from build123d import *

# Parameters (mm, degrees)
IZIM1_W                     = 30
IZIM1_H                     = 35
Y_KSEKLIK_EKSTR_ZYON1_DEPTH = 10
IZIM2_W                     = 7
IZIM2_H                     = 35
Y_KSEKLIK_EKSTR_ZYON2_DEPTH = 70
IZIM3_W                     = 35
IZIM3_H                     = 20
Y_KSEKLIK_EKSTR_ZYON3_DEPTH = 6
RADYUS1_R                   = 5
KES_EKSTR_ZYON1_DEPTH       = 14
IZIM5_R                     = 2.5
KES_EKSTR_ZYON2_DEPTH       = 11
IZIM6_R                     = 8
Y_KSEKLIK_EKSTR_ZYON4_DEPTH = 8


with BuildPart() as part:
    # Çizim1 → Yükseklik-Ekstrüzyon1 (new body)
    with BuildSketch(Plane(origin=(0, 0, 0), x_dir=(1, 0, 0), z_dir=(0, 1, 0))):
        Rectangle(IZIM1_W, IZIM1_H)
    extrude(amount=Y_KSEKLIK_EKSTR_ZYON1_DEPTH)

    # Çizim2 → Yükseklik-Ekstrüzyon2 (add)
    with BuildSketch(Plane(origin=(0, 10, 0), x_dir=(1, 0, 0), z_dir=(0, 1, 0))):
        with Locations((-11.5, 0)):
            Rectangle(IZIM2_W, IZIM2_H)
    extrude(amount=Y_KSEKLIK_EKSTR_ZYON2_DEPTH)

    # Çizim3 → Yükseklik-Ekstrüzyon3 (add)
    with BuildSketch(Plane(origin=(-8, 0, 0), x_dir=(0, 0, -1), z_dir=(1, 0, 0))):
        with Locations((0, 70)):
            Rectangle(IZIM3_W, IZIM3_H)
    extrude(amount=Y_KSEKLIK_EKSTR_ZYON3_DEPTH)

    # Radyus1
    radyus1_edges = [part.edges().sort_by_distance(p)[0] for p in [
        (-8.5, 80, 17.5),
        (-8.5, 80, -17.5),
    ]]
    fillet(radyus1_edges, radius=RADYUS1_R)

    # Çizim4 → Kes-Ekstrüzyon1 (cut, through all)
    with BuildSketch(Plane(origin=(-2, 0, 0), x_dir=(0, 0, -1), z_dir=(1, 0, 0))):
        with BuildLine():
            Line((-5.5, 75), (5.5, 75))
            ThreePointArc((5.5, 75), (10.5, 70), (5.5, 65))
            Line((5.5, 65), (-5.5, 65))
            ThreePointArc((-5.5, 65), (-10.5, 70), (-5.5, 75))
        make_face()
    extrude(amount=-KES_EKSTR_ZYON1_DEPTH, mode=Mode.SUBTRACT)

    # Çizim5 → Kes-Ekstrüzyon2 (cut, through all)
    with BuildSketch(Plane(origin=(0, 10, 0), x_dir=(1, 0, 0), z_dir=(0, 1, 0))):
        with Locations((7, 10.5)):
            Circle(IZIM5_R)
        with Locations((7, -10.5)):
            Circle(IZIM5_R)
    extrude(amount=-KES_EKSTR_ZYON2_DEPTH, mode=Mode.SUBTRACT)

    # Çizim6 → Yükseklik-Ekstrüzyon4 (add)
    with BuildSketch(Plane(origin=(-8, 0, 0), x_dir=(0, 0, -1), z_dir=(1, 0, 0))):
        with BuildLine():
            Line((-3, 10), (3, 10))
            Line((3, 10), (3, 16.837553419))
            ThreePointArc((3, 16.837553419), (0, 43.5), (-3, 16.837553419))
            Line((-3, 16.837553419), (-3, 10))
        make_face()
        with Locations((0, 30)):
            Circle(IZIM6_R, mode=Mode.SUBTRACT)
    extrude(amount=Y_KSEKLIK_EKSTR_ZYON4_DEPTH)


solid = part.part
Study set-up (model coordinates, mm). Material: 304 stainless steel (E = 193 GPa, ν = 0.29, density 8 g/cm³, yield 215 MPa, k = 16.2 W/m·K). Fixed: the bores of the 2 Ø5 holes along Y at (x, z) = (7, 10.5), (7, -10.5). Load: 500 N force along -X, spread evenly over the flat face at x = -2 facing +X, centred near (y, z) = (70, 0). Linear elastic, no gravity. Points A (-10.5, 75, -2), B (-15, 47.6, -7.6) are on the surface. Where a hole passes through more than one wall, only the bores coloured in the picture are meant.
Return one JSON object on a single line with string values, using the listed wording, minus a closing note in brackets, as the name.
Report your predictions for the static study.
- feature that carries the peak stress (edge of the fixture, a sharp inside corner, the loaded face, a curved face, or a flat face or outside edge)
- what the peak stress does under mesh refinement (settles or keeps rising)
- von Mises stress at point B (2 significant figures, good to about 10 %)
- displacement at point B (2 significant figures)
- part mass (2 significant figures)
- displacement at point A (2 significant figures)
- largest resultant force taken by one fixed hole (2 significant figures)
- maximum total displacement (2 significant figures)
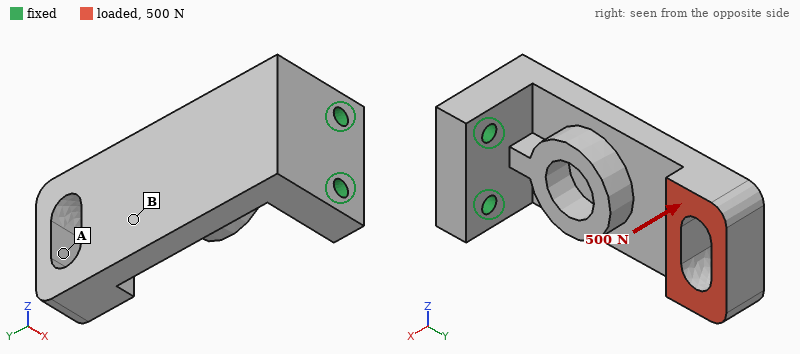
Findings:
{"feature that carries the peak stress": "edge of the fixture", "what the peak stress does under mesh refinement": "keeps rising", "von Mises stress at point B": "36 MPa", "displacement at point B": "0.072 mm", "part mass": "260 g", "displacement at point A": "0.15 mm", "largest resultant force taken by one fixed hole": "340 N", "maximum total displacement": "0.17 mm"}
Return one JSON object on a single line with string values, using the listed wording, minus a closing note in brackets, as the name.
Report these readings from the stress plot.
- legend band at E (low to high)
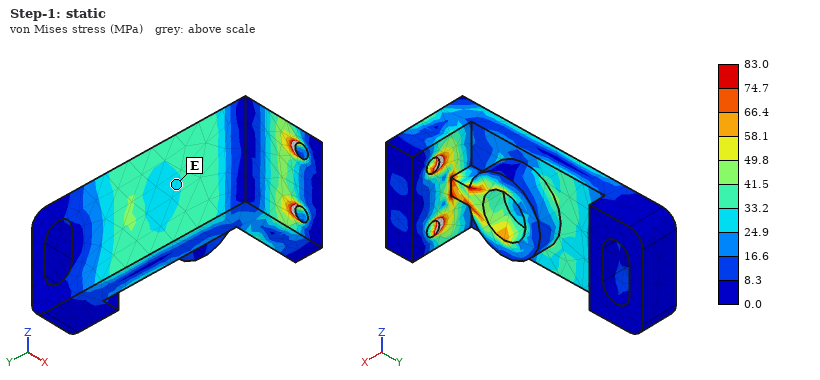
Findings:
{"legend band at E": "24.9 to 33.2 MPa"}
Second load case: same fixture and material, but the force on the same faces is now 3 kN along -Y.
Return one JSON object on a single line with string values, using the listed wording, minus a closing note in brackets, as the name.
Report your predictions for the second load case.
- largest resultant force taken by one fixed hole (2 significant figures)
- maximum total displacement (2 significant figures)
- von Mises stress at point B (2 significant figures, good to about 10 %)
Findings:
{"largest resultant force taken by one fixed hole": "1.5 kN", "maximum total displacement": "0.18 mm", "von Mises stress at point B": "82 MPa"}
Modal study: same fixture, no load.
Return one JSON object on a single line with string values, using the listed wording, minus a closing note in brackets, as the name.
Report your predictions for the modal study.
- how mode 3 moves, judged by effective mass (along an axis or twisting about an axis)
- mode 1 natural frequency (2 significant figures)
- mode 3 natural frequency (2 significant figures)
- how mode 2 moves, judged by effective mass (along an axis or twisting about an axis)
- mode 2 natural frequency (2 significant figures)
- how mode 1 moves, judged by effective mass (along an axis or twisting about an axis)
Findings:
{"how mode 3 moves, judged by effective mass": "twisting about Y", "mode 1 natural frequency": "1100 Hz", "mode 3 natural frequency": "4500 Hz", "how mode 2 moves, judged by effective mass": "along Z", "mode 2 natural frequency": "2100 Hz", "how mode 1 moves, judged by effective mass": "along X"}
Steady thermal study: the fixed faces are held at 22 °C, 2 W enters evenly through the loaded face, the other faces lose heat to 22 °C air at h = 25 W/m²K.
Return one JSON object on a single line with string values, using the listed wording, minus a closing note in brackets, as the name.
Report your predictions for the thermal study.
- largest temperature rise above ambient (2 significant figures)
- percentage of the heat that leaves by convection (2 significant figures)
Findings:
{"largest temperature rise above ambient": "16 K", "percentage of the heat that leaves by convection": "75 %"}
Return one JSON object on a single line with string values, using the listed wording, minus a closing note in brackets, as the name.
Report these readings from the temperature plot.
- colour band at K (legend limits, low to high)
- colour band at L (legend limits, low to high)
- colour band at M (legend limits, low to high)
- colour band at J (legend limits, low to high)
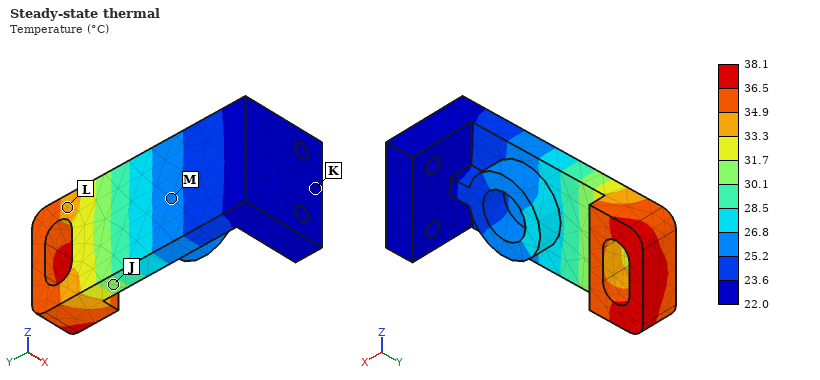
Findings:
{"colour band at K": "22.0 to 23.6 °C", "colour band at L": "33.3 to 34.9 °C", "colour band at M": "25.2 to 26.8 °C", "colour band at J": "30.1 to 31.7 °C"}
